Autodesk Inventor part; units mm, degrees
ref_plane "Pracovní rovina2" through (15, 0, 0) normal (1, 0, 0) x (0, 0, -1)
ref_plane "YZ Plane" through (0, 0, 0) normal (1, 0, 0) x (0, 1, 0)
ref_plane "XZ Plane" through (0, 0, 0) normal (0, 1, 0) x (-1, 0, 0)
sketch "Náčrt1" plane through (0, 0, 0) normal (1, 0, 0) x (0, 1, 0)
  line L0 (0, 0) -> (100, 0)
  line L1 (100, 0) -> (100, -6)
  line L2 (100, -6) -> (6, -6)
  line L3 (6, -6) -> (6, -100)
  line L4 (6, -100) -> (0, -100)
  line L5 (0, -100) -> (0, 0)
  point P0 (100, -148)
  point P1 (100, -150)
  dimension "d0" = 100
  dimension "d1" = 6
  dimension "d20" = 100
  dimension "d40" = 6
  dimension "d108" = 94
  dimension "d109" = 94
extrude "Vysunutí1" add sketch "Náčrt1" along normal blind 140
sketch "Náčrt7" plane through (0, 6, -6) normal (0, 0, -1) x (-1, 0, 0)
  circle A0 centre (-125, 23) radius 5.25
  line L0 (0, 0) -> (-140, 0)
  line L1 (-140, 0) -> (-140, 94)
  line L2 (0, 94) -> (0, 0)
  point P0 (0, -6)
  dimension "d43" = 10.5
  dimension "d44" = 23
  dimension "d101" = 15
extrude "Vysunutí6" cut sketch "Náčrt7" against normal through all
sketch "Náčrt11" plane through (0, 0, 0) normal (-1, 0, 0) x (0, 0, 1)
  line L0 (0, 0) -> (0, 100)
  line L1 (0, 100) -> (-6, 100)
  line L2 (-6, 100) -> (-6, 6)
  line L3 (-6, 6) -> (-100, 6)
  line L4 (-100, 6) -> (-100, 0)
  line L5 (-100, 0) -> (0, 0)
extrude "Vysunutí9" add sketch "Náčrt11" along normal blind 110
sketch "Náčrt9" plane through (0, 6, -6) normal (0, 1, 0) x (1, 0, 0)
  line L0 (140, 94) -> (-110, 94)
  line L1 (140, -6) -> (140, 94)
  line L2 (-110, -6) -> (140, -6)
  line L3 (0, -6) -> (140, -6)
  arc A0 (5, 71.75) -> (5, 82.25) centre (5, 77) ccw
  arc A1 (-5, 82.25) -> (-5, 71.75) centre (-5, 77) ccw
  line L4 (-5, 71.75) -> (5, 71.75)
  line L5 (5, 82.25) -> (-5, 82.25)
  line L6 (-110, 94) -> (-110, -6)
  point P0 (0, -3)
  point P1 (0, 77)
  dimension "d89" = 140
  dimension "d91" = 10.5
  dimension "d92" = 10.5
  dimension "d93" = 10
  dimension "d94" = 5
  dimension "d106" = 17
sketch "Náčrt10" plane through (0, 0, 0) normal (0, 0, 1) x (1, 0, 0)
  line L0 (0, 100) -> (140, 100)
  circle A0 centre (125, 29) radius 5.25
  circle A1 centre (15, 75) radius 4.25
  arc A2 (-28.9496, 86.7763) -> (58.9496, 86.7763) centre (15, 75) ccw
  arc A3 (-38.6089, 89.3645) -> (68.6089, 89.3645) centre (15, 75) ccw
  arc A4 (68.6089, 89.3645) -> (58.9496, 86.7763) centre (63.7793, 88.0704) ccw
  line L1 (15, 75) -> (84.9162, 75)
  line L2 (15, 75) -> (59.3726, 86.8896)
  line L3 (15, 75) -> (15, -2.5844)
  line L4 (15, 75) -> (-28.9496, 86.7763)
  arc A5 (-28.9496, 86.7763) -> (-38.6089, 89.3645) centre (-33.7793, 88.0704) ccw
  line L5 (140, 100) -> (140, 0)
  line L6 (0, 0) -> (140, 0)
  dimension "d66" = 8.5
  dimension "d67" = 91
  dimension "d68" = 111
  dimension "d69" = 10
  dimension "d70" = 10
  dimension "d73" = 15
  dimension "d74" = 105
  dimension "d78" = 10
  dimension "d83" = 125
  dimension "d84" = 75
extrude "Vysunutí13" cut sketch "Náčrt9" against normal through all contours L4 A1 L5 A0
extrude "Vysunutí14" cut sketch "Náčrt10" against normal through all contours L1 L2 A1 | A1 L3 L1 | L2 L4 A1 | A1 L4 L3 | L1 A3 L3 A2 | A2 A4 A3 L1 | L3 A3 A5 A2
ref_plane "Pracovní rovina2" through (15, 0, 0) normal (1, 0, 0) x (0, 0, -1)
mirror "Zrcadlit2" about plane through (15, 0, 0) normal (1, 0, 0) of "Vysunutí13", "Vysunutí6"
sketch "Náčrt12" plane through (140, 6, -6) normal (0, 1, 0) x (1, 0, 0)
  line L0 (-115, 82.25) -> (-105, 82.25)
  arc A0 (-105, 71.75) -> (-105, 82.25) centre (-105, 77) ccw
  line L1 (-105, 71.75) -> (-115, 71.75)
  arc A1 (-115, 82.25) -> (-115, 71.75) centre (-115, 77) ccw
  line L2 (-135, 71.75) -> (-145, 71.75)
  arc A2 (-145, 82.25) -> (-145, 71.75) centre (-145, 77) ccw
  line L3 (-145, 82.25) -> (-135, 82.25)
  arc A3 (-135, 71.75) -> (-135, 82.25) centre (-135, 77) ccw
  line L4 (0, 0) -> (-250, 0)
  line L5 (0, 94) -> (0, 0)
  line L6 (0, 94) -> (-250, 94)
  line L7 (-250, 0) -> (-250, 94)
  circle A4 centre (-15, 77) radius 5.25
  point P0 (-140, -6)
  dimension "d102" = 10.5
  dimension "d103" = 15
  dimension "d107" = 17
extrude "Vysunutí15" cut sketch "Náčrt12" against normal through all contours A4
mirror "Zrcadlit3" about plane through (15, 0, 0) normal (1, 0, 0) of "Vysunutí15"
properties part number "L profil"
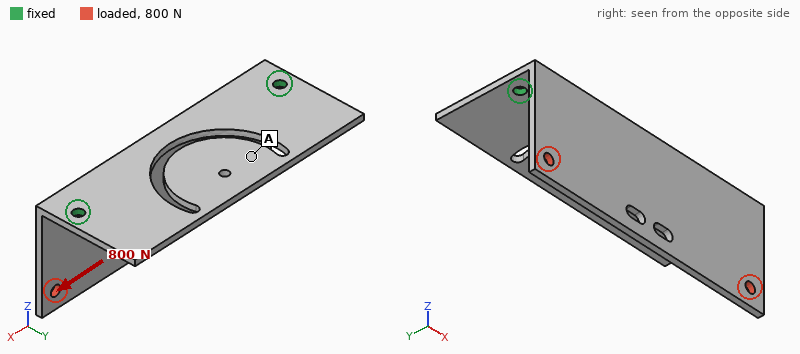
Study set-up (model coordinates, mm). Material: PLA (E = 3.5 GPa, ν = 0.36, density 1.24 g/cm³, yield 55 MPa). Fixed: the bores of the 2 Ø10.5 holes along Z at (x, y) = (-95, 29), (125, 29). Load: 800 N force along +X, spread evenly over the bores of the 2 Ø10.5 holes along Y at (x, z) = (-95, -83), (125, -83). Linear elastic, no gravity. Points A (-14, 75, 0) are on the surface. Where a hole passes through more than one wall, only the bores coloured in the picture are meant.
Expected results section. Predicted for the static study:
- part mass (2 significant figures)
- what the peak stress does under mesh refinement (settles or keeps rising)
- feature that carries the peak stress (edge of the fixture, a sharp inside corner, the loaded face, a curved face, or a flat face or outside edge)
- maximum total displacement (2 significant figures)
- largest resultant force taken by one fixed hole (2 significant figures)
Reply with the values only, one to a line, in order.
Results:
340 g
keeps rising
edge of the fixture
1.4 mm
500 N
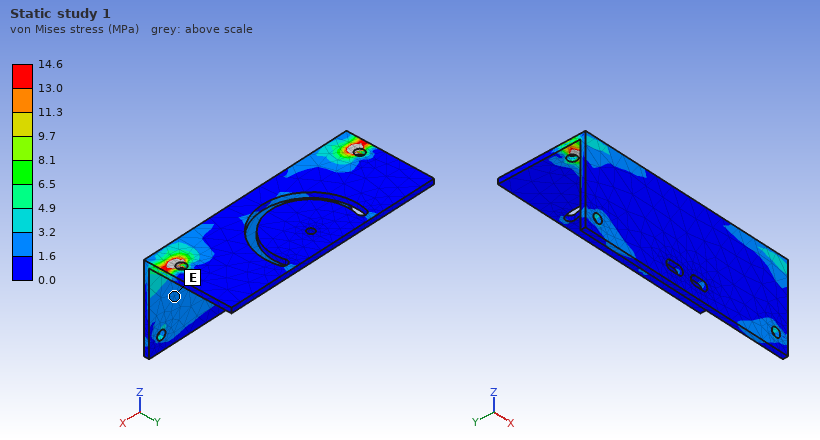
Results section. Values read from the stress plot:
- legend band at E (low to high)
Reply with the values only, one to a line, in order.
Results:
1.6 to 3.2 MPa
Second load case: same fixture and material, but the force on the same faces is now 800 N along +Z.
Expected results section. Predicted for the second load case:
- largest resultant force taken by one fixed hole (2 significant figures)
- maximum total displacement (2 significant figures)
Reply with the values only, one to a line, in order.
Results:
400 N
3.1 mm
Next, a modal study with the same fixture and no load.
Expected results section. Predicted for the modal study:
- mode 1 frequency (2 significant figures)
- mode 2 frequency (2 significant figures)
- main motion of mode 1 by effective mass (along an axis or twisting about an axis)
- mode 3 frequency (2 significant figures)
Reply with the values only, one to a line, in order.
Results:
98 Hz
130 Hz
along Y
190 Hz
